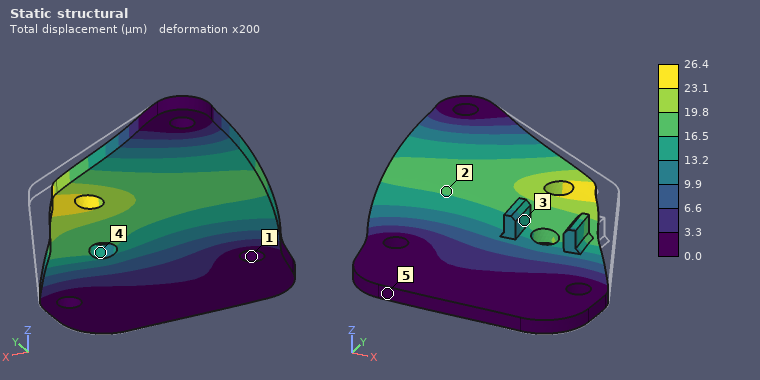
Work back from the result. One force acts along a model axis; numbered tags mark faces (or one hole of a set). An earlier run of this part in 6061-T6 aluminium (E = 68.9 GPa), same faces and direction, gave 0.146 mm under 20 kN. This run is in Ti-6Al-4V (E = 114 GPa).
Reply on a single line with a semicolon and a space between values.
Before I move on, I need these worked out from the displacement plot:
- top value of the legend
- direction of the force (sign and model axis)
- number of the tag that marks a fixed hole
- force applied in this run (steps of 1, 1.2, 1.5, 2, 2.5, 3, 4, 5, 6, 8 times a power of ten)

26.4 µm; -X; 1; 6 kN
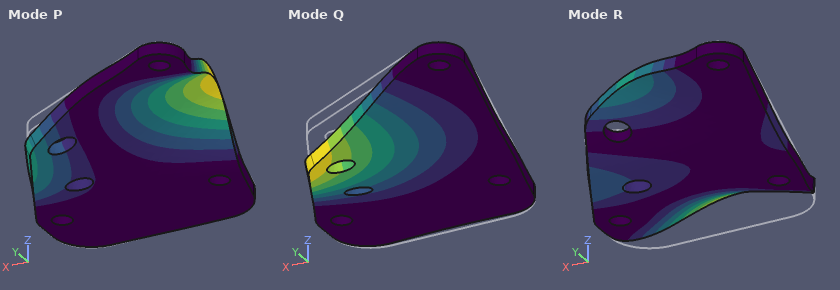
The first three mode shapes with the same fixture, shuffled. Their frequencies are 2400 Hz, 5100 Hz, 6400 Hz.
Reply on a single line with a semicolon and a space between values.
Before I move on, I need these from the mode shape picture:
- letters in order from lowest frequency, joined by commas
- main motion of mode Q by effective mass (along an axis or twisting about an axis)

Q, P, R; along Z
